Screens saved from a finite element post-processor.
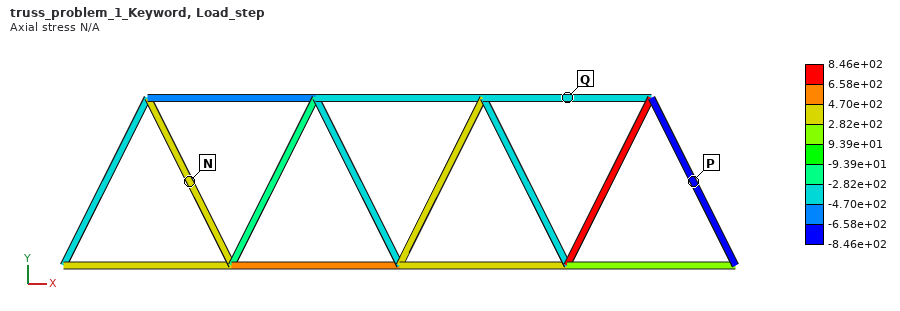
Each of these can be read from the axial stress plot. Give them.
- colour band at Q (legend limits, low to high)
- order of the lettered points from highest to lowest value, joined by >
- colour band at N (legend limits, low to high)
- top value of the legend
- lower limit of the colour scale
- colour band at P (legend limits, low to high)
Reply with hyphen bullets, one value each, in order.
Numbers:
- -4.70e+02 to -2.82e+02
- N > Q > P
- 2.82e+02 to 4.70e+02
- 8.46e+02
- -8.46e+02
- -8.46e+02 to -6.58e+02
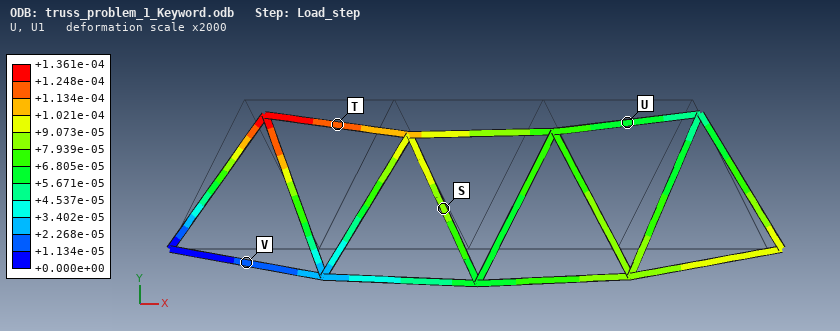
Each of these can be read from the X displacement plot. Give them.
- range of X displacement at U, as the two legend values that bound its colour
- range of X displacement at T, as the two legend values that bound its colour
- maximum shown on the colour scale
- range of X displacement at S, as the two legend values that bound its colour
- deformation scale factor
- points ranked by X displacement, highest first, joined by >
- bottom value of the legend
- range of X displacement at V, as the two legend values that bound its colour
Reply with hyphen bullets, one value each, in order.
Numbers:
- +5.671e-05 to +6.805e-05
- +1.134e-04 to +1.248e-04
- +1.361e-04
- +7.939e-05 to +9.073e-05
- 2000
- T > S > U > V
- +0.000e+00
- +1.134e-05 to +2.268e-05
